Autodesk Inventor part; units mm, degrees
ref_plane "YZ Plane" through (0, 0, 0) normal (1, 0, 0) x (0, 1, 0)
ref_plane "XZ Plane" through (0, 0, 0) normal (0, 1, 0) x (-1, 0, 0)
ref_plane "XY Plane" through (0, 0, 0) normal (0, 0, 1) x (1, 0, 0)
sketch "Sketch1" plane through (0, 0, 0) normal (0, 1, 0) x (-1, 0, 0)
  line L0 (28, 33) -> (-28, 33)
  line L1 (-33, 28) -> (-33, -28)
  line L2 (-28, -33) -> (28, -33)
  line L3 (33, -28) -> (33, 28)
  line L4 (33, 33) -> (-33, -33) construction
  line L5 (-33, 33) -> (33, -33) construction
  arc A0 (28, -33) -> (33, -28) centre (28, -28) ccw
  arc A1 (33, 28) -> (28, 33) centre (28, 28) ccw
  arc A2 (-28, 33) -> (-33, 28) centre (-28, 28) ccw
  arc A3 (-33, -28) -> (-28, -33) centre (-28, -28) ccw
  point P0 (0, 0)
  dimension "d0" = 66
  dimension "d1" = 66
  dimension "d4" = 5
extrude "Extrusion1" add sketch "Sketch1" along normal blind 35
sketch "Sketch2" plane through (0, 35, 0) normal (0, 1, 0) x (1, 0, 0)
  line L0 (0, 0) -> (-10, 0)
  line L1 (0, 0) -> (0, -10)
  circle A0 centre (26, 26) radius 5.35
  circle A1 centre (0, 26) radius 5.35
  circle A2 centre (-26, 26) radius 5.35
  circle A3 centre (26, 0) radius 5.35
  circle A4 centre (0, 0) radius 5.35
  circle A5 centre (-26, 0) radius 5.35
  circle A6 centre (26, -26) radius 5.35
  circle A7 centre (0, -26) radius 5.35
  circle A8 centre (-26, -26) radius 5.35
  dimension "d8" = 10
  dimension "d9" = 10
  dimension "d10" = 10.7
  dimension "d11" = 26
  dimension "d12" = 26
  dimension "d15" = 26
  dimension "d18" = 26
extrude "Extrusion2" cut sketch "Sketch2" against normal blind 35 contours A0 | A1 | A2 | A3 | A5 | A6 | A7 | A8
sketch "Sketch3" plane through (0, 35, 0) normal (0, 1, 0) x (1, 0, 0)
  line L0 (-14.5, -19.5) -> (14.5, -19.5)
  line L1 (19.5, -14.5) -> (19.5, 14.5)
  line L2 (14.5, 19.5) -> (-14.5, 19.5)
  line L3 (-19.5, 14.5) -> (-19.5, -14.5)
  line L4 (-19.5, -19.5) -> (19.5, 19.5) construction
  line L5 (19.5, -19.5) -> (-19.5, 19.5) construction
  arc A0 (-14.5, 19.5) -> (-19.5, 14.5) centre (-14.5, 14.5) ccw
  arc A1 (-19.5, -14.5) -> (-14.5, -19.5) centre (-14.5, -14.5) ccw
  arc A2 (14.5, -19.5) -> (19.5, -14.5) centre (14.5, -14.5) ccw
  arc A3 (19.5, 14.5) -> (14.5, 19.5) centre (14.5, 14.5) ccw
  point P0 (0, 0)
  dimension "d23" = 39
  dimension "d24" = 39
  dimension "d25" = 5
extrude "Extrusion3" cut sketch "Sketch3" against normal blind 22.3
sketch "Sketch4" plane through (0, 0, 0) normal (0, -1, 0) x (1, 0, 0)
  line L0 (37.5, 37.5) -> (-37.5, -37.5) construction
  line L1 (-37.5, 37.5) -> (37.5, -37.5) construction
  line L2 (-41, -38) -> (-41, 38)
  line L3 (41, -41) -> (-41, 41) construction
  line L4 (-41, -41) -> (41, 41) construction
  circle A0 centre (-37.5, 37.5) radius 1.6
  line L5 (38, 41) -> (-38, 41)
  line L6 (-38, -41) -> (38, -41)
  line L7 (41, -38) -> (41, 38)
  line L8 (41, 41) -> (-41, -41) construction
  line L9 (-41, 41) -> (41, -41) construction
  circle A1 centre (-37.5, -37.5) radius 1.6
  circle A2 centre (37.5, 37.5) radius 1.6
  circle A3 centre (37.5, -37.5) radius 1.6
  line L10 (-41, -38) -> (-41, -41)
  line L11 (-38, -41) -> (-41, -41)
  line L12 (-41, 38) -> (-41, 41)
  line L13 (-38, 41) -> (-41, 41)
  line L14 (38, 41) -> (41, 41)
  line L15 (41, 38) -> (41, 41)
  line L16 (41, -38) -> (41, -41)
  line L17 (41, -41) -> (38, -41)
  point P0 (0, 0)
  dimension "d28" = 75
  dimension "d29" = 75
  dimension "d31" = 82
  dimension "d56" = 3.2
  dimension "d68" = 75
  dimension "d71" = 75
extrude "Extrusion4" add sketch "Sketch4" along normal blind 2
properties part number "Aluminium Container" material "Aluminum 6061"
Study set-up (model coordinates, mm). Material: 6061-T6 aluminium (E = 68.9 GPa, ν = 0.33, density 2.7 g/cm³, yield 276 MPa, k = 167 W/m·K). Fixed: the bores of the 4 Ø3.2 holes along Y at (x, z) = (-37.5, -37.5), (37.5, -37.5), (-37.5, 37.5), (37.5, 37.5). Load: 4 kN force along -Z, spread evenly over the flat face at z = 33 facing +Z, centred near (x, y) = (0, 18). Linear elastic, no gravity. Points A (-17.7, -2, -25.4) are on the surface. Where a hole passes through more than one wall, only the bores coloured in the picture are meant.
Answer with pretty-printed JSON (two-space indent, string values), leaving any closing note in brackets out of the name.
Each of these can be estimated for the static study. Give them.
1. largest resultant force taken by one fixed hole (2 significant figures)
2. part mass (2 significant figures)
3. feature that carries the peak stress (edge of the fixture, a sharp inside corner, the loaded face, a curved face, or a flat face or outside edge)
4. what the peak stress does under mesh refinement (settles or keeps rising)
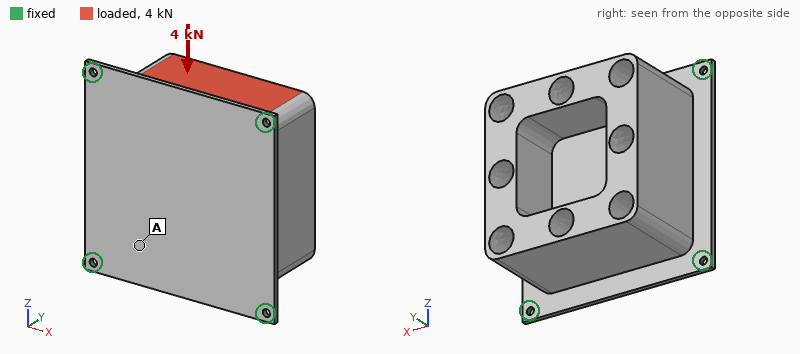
{
  "largest resultant force taken by one fixed hole": "1.2 kN",
  "part mass": "290 g",
  "feature that carries the peak stress": "edge of the fixture",
  "what the peak stress does under mesh refinement": "keeps rising"
}
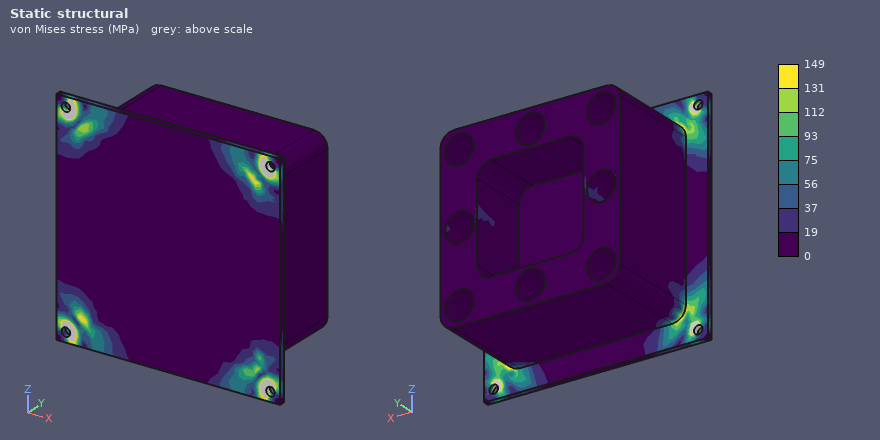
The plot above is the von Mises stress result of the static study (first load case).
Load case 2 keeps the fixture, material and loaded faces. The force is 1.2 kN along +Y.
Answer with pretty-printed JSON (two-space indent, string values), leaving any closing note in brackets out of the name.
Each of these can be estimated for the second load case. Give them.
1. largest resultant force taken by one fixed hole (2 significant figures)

{
  "largest resultant force taken by one fixed hole": "620 N"
}
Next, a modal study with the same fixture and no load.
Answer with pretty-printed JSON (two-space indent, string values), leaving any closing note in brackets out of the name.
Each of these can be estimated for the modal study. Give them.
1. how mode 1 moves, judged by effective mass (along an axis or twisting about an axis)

{
  "how mode 1 moves, judged by effective mass": "along Y"
}
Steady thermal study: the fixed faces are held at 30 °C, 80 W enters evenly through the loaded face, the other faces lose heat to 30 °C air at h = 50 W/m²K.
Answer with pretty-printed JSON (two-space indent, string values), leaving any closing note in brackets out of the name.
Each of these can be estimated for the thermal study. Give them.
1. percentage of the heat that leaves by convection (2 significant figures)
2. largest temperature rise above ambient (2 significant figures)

{
  "percentage of the heat that leaves by convection": "52 %",
  "largest temperature rise above ambient": "38 K"
}
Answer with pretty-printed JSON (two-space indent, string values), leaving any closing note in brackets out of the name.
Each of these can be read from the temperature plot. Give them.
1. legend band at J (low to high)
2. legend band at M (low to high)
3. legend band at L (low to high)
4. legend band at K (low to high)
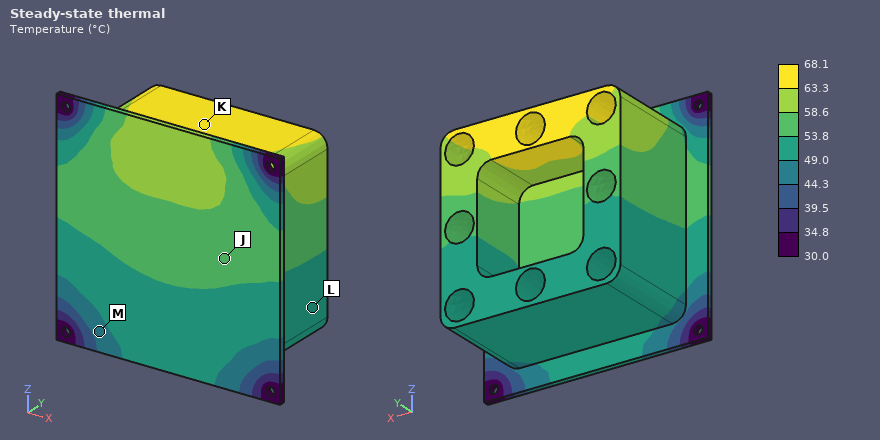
{
  "legend band at J": "53.8 to 58.6 °C",
  "legend band at M": "44.3 to 49.0 °C",
  "legend band at L": "49.0 to 53.8 °C",
  "legend band at K": "63.3 to 68.1 °C"
}
